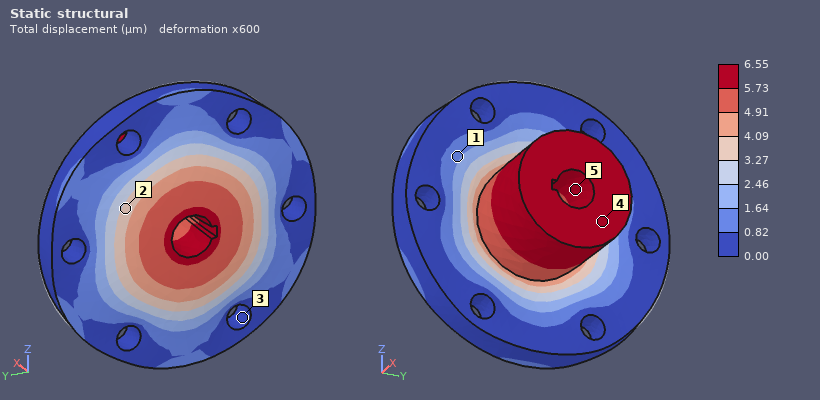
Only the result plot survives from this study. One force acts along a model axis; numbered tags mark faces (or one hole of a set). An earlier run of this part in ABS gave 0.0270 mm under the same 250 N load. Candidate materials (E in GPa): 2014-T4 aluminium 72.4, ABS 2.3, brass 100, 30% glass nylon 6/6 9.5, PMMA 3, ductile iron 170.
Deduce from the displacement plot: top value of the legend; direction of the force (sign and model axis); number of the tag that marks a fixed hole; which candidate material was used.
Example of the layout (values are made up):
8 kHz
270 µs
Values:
6.55 µm
-X
3
30% glass nylon 6/6
